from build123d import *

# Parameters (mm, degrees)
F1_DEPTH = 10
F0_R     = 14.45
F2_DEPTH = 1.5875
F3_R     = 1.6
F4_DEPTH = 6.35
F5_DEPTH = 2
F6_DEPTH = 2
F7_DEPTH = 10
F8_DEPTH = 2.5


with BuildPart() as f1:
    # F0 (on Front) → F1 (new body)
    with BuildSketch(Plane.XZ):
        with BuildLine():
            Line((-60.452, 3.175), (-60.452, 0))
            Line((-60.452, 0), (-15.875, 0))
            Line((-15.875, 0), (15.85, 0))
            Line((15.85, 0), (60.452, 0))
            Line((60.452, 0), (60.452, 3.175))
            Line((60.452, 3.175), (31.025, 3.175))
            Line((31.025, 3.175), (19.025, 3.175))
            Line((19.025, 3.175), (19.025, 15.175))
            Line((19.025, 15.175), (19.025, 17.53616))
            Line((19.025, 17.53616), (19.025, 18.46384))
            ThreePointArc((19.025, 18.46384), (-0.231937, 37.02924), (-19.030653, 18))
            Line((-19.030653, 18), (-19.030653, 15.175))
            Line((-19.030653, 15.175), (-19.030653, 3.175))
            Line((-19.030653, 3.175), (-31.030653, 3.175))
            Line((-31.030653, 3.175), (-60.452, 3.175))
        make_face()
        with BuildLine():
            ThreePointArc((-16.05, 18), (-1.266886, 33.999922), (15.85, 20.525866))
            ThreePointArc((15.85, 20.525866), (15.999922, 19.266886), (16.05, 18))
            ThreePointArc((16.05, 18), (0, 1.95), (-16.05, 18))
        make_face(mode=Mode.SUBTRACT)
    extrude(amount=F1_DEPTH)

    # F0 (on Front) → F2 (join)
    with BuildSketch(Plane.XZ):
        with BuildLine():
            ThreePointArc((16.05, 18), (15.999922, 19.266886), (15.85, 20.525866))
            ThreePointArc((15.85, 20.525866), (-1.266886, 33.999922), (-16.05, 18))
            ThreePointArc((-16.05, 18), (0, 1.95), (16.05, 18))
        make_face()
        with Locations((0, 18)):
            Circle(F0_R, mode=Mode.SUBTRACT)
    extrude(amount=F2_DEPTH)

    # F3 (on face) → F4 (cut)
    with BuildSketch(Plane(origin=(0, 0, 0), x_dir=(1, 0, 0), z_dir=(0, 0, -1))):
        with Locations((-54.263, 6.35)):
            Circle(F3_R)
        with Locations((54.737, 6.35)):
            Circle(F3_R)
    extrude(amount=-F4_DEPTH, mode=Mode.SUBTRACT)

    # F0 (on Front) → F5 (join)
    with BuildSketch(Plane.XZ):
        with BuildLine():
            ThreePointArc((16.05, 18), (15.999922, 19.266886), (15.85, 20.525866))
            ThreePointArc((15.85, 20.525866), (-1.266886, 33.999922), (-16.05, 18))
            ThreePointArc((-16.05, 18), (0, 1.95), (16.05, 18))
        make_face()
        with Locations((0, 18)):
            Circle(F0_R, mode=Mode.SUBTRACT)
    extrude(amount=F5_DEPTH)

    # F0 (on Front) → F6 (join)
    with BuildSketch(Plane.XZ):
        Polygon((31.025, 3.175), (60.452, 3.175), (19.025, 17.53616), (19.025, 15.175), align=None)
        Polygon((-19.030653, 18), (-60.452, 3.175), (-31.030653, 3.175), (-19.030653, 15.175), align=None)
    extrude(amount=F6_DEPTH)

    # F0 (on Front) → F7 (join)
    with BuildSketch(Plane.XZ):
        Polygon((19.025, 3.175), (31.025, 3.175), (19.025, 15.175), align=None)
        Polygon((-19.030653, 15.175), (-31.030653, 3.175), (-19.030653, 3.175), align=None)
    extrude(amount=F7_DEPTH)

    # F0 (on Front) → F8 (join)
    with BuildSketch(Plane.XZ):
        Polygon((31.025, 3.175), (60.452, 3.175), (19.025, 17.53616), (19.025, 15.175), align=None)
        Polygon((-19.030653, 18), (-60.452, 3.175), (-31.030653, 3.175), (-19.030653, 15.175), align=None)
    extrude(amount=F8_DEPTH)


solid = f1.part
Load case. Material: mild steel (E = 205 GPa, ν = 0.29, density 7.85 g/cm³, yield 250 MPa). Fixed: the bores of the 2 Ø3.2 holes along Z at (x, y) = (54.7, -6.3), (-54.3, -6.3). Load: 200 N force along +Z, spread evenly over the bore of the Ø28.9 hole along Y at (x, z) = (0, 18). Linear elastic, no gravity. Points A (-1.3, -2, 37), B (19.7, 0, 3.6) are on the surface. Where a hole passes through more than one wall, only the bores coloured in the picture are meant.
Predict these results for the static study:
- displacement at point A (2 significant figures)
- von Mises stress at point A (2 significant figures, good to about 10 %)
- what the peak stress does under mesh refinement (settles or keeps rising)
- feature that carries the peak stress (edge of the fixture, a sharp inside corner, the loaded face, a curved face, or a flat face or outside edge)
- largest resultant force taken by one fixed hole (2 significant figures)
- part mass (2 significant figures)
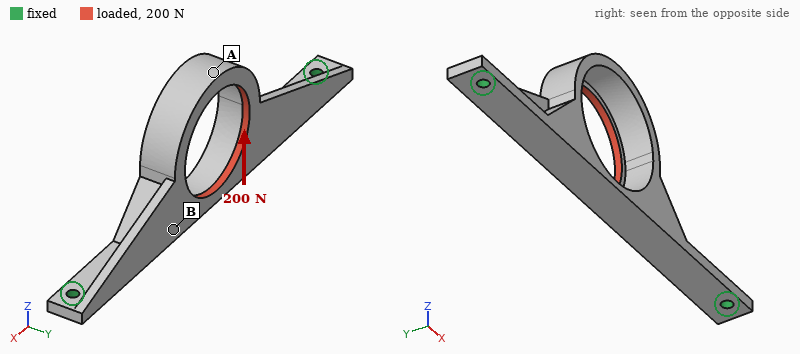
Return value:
33 µm
19 MPa
keeps rising
edge of the fixture
120 N
78 g
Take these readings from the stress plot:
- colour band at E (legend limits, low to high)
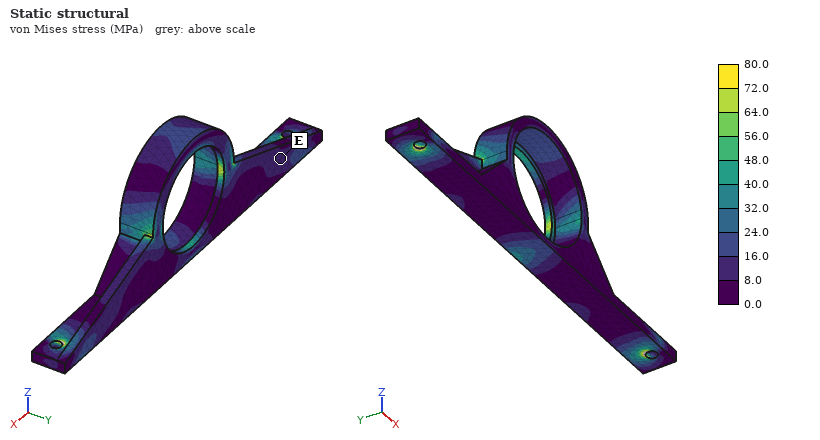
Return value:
8.0 to 16.0 MPa
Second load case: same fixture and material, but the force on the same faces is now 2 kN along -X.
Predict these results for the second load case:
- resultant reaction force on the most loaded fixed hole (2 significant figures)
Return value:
1.1 kN
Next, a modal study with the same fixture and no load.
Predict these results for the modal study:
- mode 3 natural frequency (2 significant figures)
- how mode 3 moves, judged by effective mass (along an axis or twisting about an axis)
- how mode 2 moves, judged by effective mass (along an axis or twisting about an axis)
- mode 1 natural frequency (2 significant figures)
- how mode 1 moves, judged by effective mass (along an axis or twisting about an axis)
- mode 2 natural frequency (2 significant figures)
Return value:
3300 Hz
along Y
along Z
1200 Hz
along Y
1900 Hz
